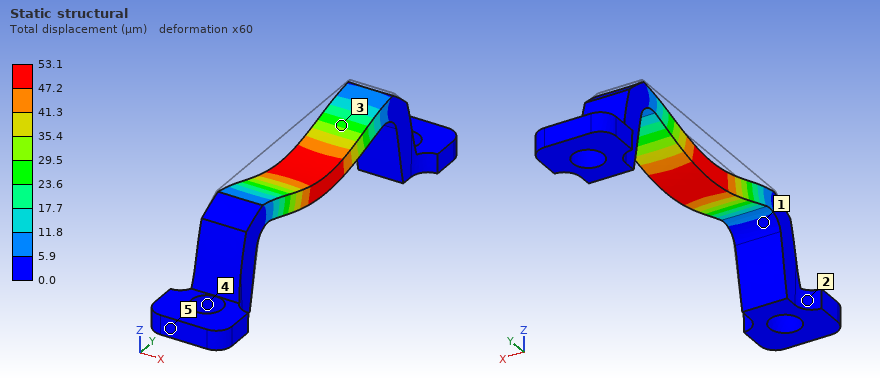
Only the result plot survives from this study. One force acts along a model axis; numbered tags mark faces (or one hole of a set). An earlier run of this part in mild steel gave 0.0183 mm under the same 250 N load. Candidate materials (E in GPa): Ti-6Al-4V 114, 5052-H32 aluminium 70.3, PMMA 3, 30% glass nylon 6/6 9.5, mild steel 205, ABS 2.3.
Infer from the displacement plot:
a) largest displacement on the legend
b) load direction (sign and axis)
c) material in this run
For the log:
53.1 µm
-Z
5052-H32 aluminium
